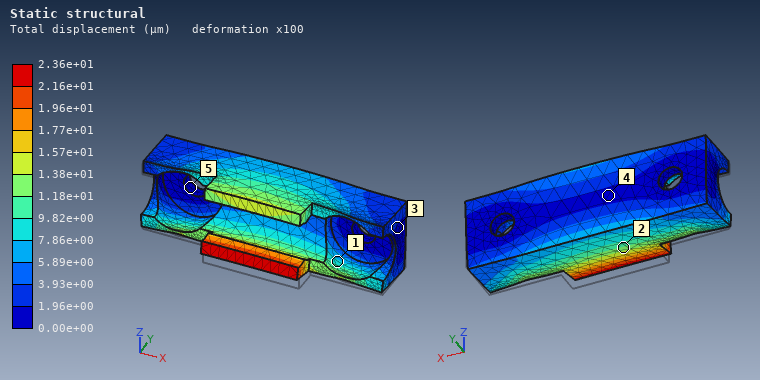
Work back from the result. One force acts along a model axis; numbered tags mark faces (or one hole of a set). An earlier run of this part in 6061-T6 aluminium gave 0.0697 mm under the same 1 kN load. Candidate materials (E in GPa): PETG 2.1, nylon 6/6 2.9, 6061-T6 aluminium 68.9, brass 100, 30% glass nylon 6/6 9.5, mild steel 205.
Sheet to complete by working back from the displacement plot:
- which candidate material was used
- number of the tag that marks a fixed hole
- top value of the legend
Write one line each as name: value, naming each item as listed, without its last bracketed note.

which candidate material was used: mild steel
number of the tag that marks a fixed hole: 5
top value of the legend: 2.36e+01 µm
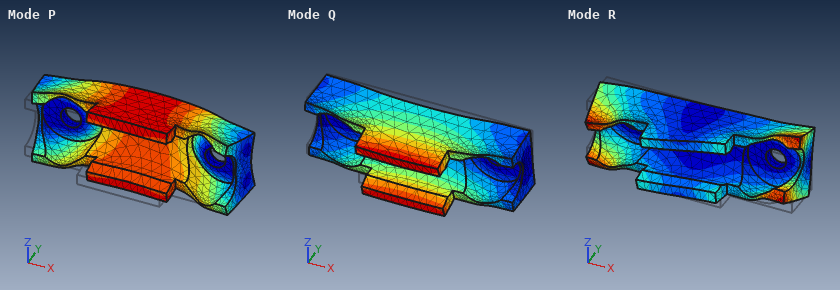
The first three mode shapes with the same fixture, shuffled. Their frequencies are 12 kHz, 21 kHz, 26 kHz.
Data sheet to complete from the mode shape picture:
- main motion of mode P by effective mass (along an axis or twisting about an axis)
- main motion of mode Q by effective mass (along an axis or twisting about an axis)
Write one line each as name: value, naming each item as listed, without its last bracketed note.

main motion of mode P by effective mass: along Y
main motion of mode Q by effective mass: along Z
